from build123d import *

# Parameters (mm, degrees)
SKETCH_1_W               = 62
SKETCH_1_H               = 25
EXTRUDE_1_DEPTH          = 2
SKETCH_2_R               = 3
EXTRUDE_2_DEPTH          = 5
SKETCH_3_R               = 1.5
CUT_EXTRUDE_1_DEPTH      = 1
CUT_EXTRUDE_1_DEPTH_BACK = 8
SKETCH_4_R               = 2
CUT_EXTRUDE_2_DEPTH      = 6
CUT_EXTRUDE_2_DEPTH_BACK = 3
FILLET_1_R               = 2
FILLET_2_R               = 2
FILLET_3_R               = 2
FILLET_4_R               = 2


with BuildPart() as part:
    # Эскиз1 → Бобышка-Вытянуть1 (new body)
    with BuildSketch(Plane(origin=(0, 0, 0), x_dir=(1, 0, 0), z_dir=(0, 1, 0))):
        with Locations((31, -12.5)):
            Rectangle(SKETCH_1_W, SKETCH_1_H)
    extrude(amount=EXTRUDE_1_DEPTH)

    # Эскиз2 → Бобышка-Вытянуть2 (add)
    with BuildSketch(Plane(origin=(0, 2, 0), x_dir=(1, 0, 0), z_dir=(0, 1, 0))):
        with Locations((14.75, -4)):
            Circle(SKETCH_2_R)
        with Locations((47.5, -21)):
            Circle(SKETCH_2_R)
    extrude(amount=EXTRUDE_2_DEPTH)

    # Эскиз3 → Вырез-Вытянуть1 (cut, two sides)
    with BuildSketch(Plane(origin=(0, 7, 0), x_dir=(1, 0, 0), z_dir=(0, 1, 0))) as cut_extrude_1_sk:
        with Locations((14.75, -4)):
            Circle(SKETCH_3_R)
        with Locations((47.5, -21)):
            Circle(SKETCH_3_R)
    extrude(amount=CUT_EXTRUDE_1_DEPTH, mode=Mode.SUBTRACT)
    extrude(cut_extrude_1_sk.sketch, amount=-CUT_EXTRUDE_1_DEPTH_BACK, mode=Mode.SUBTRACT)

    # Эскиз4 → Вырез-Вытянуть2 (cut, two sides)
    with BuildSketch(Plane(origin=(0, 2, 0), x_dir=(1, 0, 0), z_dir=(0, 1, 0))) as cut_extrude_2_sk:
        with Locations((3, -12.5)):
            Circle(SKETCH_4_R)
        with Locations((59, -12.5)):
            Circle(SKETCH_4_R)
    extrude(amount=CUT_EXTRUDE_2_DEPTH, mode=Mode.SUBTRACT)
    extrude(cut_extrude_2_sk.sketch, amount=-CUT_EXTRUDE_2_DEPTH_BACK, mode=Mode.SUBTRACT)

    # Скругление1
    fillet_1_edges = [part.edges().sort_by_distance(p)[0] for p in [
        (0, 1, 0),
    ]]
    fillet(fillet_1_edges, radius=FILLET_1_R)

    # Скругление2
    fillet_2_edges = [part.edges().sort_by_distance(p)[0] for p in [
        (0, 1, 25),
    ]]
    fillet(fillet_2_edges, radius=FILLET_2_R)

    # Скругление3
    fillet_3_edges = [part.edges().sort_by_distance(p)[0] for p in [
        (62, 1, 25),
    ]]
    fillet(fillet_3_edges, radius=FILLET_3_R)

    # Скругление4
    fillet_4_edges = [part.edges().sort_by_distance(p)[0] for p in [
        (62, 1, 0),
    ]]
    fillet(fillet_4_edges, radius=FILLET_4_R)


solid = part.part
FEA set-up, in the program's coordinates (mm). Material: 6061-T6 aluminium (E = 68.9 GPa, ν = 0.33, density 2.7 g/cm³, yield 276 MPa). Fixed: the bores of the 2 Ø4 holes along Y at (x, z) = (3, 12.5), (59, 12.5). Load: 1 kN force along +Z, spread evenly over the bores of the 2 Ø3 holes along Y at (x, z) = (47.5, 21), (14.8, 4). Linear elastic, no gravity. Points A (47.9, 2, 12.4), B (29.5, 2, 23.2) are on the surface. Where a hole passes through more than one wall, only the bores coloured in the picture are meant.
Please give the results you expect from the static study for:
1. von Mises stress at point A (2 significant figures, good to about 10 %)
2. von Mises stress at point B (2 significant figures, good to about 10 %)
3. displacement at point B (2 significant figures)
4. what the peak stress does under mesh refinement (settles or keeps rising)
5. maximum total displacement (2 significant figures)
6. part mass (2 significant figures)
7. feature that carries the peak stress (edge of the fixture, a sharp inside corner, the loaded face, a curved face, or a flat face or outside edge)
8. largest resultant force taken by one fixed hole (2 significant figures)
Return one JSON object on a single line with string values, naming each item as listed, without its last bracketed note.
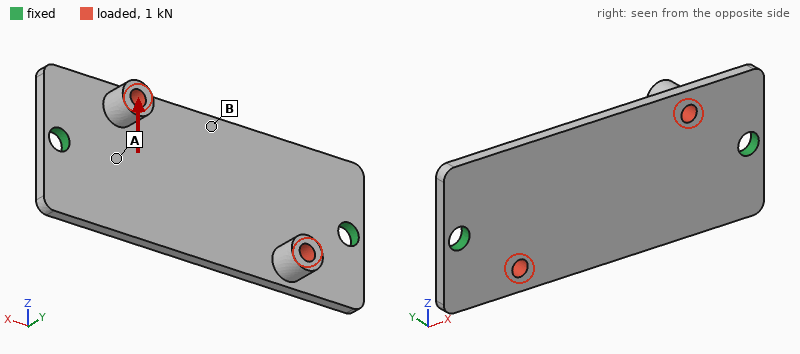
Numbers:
{"von Mises stress at point A": "63 MPa", "von Mises stress at point B": "22 MPa", "displacement at point B": "0.10 mm", "what the peak stress does under mesh refinement": "keeps rising", "maximum total displacement": "0.16 mm", "part mass": "8.7 g", "feature that carries the peak stress": "edge of the fixture", "largest resultant force taken by one fixed hole": "500 N"}
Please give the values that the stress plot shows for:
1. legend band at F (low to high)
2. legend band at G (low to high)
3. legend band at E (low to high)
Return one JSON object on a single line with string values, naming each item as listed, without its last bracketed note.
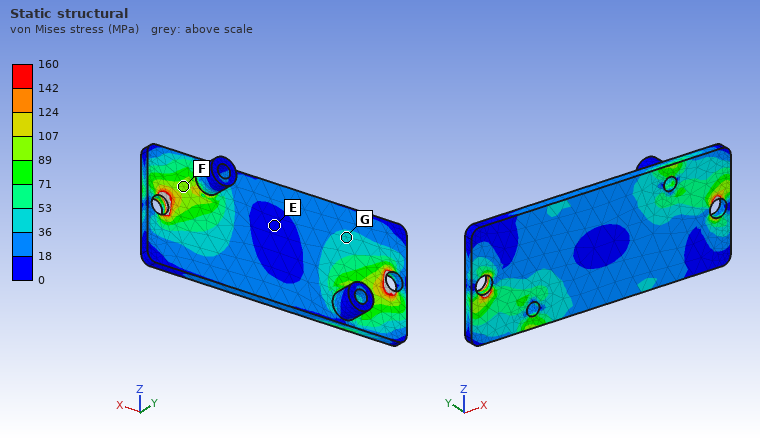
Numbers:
{"legend band at F": "89 to 107 MPa", "legend band at G": "36 to 53 MPa", "legend band at E": "0 to 18 MPa"}
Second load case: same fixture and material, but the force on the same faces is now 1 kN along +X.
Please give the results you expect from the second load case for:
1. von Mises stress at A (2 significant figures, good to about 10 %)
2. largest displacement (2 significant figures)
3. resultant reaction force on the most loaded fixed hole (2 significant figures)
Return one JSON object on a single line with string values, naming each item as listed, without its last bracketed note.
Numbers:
{"von Mises stress at A": "35 MPa", "largest displacement": "75 µm", "resultant reaction force on the most loaded fixed hole": "500 N"}
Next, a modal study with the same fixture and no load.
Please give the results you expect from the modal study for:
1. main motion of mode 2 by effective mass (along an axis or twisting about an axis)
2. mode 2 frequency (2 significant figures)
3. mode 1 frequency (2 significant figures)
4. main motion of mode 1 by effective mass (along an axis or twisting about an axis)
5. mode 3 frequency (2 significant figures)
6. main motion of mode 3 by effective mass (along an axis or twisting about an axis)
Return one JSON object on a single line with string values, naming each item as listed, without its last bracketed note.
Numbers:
{"main motion of mode 2 by effective mass": "twisting about X", "mode 2 frequency": "4100 Hz", "mode 1 frequency": "3100 Hz", "main motion of mode 1 by effective mass": "along Y", "mode 3 frequency": "7900 Hz", "main motion of mode 3 by effective mass": "twisting about Z"}
